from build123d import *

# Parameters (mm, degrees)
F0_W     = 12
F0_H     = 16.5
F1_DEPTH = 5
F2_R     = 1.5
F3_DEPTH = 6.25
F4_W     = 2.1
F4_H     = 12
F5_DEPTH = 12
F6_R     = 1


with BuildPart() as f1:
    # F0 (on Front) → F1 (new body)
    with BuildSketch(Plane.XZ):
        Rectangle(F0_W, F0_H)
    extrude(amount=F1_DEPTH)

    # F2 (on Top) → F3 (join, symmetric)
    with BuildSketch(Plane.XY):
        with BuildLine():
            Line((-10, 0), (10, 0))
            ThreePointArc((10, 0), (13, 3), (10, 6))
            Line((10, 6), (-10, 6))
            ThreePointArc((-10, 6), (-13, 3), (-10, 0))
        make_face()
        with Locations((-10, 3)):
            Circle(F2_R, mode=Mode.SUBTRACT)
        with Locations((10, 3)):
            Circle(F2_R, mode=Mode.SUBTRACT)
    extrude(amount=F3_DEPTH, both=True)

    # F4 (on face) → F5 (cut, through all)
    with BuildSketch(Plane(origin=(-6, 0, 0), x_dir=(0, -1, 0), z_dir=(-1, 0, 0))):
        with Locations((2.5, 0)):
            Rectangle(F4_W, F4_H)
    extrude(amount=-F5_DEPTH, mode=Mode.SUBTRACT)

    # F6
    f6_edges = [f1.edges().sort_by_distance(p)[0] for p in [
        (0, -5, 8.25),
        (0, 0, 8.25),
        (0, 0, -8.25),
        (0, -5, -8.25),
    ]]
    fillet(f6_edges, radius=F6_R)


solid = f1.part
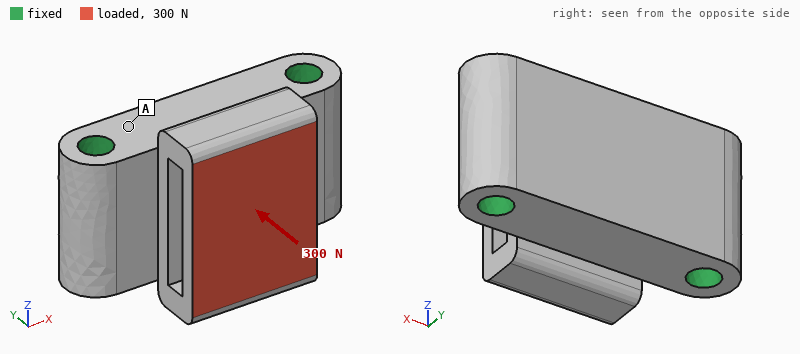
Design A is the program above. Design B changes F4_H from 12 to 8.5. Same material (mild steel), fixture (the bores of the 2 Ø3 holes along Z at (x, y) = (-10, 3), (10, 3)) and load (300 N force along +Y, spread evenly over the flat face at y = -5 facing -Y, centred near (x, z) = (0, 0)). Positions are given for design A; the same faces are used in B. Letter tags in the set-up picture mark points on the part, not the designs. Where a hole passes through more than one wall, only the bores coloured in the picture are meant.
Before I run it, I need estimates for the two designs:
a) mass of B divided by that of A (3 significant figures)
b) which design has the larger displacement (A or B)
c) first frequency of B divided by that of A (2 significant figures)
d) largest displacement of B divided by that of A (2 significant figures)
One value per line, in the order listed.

1.04
A
1.2
0.34
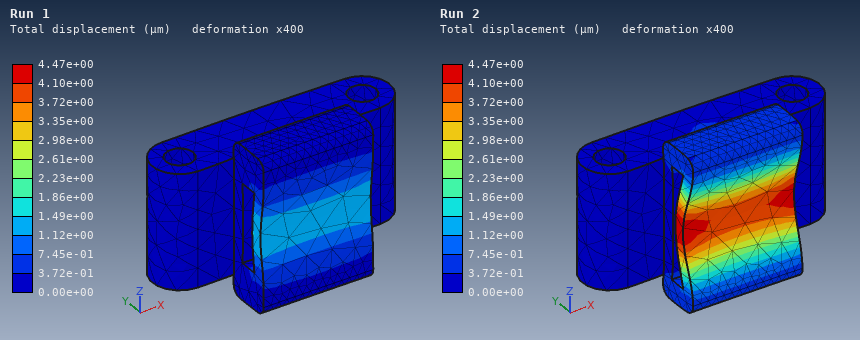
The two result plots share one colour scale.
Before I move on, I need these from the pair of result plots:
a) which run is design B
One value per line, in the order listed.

Run 1
